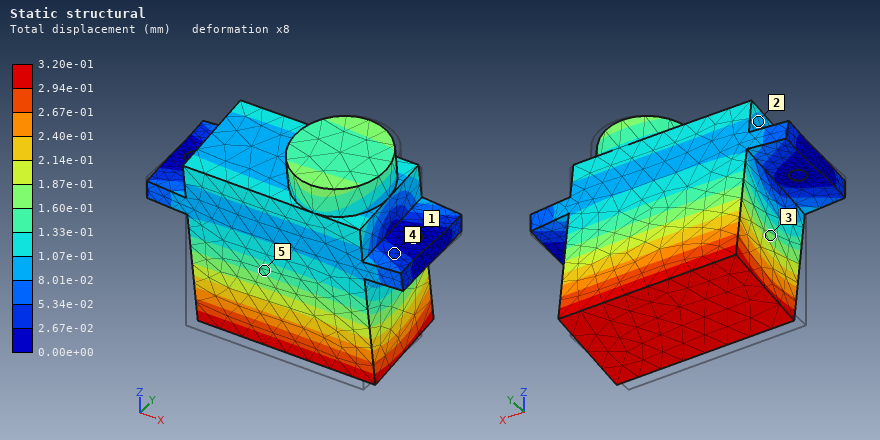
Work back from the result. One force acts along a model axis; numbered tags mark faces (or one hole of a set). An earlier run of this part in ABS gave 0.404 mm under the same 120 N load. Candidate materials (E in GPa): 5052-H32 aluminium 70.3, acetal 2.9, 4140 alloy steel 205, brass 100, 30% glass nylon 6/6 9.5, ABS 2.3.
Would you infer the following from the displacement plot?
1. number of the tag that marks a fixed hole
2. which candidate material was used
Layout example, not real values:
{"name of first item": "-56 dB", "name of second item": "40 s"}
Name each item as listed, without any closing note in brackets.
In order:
{"number of the tag that marks a fixed hole": "1", "which candidate material was used": "acetal"}
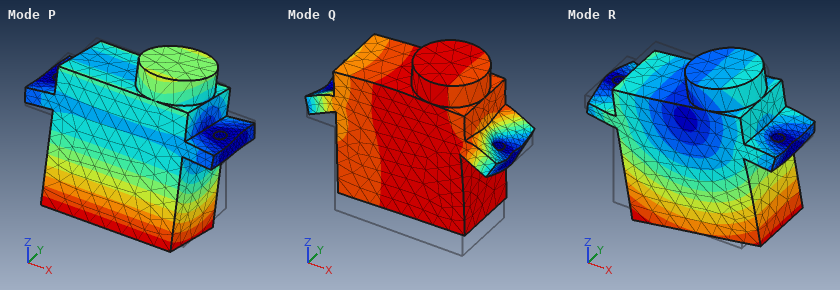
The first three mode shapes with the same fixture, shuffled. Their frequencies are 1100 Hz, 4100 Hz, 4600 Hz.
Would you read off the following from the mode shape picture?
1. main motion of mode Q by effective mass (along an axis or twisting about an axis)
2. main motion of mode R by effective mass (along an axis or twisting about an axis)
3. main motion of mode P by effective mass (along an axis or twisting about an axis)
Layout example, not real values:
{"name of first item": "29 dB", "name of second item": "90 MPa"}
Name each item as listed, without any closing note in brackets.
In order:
{"main motion of mode Q by effective mass": "along Z", "main motion of mode R by effective mass": "along X", "main motion of mode P by effective mass": "along Y"}
